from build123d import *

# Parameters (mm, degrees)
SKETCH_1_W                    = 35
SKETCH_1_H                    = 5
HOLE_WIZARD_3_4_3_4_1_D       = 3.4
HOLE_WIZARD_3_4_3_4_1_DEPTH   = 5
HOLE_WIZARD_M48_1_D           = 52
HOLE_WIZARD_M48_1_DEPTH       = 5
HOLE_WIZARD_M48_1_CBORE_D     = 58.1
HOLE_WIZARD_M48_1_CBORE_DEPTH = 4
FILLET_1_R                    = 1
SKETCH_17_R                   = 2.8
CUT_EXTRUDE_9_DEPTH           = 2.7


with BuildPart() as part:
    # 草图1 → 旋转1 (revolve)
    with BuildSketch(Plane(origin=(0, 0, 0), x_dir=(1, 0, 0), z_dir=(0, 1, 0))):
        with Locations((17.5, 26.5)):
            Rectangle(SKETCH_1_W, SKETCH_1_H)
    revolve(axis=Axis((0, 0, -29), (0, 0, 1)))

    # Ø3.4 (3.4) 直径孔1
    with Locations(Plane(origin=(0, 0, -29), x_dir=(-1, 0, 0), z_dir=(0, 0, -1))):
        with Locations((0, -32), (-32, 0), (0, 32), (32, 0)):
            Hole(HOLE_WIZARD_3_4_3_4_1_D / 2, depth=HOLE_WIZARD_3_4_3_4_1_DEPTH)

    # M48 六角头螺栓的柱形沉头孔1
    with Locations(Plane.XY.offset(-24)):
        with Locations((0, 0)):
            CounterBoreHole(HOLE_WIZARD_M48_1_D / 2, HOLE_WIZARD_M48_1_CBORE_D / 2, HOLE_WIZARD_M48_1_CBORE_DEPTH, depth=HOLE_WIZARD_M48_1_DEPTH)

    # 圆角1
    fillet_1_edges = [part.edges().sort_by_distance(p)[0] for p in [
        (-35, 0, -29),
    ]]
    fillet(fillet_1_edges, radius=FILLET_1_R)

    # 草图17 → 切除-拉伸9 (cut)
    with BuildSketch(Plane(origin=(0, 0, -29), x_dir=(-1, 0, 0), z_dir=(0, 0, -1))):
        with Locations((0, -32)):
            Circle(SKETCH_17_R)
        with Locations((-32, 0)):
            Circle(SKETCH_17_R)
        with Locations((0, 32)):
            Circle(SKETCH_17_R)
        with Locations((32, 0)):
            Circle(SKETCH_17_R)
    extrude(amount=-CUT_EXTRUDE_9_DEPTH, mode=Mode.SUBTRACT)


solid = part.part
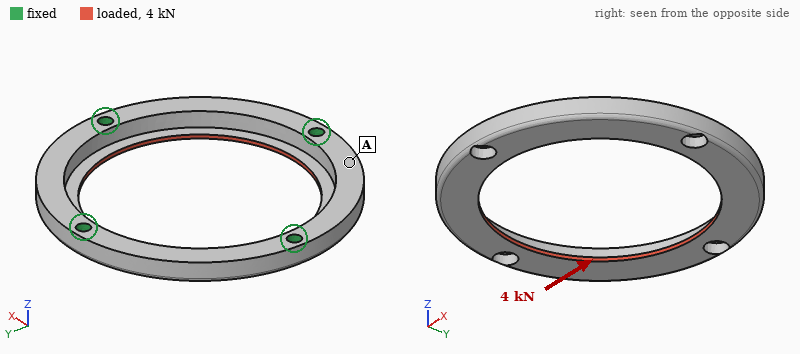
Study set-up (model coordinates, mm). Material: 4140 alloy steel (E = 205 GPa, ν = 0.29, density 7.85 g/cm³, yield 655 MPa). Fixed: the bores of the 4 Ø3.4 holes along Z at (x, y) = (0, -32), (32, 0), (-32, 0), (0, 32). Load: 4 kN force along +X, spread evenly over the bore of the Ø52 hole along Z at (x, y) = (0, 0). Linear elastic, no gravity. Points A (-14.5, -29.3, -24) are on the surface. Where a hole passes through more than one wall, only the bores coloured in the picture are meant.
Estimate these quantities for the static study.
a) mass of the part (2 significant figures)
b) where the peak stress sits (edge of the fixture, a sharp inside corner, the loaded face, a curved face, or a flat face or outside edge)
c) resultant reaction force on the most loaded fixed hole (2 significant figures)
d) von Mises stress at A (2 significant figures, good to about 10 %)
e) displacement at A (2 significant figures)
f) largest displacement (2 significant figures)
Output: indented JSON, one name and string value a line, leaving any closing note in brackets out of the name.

{
  "mass of the part": "48 g",
  "where the peak stress sits": "a curved face",
  "resultant reaction force on the most loaded fixed hole": "1.4 kN",
  "von Mises stress at A": "27 MPa",
  "displacement at A": "8.8 µm",
  "largest displacement": "15 µm"
}
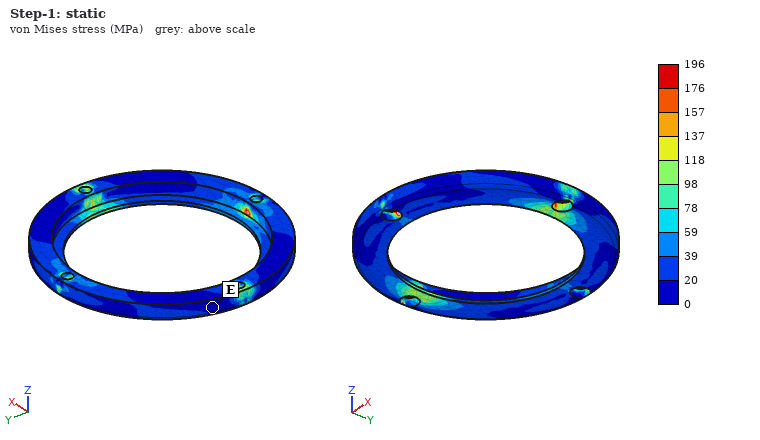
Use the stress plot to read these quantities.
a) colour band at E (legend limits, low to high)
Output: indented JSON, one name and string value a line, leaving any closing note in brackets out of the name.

{
  "colour band at E": "0 to 20 MPa"
}
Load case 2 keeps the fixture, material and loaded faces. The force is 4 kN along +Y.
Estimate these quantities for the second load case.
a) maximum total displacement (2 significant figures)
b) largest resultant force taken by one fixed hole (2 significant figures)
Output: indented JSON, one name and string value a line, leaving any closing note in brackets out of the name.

{
  "maximum total displacement": "15 µm",
  "largest resultant force taken by one fixed hole": "1.4 kN"
}
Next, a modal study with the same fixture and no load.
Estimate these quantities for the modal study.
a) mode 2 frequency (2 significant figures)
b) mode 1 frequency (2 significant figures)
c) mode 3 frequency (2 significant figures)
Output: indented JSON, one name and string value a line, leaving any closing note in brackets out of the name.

{
  "mode 2 frequency": "7600 Hz",
  "mode 1 frequency": "6500 Hz",
  "mode 3 frequency": "7600 Hz"
}
